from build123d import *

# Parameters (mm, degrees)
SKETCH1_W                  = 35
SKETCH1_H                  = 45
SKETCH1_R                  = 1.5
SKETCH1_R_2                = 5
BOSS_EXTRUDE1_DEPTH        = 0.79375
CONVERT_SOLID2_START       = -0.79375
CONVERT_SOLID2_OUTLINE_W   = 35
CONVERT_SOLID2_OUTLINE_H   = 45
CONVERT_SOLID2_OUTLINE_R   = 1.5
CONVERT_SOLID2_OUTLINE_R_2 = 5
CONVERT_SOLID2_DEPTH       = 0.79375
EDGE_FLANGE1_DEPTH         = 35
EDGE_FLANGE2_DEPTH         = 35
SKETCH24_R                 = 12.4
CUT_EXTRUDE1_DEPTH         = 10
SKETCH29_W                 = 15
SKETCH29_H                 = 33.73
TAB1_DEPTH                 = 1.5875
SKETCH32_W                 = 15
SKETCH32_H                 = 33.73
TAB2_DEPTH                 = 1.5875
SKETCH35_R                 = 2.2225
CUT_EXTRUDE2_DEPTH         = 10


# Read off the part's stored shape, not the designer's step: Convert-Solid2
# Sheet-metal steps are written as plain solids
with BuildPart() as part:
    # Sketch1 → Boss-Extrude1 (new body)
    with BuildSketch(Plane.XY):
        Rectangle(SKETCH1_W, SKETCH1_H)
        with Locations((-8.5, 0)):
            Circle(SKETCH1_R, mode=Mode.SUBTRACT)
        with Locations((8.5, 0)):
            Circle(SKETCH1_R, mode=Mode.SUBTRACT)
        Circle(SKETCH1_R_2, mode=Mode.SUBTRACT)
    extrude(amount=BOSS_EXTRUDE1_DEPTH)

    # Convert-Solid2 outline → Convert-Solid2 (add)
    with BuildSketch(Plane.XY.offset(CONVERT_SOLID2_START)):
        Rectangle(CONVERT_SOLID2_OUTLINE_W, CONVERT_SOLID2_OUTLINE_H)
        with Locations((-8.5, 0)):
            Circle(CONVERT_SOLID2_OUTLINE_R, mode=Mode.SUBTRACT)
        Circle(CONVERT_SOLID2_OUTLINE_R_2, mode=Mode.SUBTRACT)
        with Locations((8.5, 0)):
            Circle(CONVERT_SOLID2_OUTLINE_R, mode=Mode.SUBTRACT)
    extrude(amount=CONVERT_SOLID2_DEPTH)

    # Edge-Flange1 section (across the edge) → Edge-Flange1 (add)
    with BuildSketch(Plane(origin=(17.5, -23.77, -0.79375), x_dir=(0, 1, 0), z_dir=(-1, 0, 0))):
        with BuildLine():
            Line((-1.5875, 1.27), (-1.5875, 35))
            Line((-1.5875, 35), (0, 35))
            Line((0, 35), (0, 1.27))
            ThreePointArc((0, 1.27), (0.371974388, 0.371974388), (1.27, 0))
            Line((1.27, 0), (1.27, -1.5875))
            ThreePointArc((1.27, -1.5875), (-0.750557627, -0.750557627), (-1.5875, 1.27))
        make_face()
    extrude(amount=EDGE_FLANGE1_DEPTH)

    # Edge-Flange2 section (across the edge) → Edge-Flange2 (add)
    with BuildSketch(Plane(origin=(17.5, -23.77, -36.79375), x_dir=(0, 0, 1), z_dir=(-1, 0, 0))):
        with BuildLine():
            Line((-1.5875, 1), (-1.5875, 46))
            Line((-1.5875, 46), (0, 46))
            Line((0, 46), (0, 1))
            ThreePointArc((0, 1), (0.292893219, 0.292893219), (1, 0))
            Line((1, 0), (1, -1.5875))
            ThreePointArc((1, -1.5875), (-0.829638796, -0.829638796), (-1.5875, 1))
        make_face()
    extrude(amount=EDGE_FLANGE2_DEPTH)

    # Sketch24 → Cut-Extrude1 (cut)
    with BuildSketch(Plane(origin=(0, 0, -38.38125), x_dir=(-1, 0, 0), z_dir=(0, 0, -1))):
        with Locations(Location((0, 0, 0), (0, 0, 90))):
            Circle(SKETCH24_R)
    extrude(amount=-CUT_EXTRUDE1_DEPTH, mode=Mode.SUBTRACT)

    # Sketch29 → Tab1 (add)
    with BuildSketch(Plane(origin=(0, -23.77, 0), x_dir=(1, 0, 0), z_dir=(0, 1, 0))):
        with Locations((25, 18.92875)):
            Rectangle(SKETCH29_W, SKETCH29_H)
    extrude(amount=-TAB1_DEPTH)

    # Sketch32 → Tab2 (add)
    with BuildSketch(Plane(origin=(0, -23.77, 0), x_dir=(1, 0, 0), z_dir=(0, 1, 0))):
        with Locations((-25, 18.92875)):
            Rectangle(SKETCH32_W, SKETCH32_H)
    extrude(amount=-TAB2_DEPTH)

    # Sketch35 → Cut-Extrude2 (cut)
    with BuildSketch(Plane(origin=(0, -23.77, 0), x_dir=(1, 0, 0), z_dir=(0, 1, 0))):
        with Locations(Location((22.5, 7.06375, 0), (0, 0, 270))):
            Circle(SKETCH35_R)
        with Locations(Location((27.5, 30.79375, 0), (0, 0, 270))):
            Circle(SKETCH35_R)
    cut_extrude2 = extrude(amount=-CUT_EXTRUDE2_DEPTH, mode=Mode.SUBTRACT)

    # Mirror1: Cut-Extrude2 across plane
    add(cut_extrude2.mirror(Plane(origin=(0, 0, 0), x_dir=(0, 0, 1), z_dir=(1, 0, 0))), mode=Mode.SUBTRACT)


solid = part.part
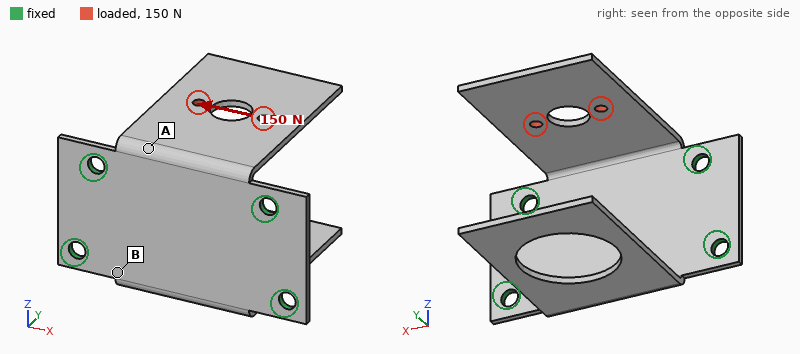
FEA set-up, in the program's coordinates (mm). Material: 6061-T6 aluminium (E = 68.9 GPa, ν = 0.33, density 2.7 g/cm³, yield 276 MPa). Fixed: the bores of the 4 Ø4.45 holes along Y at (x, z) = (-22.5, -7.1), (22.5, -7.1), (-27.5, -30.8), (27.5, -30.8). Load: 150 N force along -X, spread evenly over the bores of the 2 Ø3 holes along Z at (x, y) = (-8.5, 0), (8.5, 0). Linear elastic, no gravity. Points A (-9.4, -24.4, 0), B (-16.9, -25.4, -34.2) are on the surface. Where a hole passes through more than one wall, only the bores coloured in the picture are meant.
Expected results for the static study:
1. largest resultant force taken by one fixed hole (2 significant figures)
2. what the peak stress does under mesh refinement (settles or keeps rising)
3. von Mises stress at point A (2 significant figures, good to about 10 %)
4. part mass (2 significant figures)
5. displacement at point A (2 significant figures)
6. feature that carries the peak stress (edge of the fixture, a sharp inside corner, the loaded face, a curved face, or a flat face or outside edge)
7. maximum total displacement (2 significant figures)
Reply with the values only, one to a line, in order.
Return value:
130 N
keeps rising
27 MPa
21 g
0.030 mm
a sharp inside corner
0.18 mm
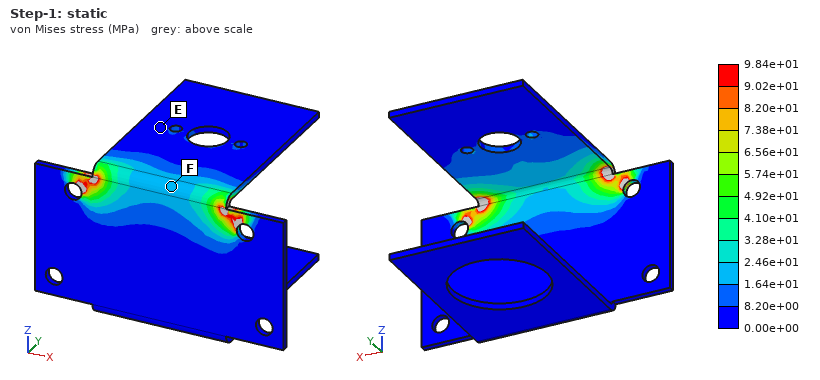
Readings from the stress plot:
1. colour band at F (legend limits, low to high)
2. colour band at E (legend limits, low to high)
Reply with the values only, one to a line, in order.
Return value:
1.64e+01 to 2.46e+01 MPa
0.00e+00 to 8.20e+00 MPa
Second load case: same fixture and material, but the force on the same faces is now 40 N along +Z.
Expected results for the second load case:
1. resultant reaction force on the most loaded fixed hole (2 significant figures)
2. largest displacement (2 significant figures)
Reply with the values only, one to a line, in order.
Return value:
18 N
0.98 mm
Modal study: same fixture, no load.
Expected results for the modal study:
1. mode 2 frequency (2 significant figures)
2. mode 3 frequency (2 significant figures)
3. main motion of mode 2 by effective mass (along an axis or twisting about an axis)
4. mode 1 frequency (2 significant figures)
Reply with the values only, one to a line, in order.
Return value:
470 Hz
1400 Hz
along Z
440 Hz
